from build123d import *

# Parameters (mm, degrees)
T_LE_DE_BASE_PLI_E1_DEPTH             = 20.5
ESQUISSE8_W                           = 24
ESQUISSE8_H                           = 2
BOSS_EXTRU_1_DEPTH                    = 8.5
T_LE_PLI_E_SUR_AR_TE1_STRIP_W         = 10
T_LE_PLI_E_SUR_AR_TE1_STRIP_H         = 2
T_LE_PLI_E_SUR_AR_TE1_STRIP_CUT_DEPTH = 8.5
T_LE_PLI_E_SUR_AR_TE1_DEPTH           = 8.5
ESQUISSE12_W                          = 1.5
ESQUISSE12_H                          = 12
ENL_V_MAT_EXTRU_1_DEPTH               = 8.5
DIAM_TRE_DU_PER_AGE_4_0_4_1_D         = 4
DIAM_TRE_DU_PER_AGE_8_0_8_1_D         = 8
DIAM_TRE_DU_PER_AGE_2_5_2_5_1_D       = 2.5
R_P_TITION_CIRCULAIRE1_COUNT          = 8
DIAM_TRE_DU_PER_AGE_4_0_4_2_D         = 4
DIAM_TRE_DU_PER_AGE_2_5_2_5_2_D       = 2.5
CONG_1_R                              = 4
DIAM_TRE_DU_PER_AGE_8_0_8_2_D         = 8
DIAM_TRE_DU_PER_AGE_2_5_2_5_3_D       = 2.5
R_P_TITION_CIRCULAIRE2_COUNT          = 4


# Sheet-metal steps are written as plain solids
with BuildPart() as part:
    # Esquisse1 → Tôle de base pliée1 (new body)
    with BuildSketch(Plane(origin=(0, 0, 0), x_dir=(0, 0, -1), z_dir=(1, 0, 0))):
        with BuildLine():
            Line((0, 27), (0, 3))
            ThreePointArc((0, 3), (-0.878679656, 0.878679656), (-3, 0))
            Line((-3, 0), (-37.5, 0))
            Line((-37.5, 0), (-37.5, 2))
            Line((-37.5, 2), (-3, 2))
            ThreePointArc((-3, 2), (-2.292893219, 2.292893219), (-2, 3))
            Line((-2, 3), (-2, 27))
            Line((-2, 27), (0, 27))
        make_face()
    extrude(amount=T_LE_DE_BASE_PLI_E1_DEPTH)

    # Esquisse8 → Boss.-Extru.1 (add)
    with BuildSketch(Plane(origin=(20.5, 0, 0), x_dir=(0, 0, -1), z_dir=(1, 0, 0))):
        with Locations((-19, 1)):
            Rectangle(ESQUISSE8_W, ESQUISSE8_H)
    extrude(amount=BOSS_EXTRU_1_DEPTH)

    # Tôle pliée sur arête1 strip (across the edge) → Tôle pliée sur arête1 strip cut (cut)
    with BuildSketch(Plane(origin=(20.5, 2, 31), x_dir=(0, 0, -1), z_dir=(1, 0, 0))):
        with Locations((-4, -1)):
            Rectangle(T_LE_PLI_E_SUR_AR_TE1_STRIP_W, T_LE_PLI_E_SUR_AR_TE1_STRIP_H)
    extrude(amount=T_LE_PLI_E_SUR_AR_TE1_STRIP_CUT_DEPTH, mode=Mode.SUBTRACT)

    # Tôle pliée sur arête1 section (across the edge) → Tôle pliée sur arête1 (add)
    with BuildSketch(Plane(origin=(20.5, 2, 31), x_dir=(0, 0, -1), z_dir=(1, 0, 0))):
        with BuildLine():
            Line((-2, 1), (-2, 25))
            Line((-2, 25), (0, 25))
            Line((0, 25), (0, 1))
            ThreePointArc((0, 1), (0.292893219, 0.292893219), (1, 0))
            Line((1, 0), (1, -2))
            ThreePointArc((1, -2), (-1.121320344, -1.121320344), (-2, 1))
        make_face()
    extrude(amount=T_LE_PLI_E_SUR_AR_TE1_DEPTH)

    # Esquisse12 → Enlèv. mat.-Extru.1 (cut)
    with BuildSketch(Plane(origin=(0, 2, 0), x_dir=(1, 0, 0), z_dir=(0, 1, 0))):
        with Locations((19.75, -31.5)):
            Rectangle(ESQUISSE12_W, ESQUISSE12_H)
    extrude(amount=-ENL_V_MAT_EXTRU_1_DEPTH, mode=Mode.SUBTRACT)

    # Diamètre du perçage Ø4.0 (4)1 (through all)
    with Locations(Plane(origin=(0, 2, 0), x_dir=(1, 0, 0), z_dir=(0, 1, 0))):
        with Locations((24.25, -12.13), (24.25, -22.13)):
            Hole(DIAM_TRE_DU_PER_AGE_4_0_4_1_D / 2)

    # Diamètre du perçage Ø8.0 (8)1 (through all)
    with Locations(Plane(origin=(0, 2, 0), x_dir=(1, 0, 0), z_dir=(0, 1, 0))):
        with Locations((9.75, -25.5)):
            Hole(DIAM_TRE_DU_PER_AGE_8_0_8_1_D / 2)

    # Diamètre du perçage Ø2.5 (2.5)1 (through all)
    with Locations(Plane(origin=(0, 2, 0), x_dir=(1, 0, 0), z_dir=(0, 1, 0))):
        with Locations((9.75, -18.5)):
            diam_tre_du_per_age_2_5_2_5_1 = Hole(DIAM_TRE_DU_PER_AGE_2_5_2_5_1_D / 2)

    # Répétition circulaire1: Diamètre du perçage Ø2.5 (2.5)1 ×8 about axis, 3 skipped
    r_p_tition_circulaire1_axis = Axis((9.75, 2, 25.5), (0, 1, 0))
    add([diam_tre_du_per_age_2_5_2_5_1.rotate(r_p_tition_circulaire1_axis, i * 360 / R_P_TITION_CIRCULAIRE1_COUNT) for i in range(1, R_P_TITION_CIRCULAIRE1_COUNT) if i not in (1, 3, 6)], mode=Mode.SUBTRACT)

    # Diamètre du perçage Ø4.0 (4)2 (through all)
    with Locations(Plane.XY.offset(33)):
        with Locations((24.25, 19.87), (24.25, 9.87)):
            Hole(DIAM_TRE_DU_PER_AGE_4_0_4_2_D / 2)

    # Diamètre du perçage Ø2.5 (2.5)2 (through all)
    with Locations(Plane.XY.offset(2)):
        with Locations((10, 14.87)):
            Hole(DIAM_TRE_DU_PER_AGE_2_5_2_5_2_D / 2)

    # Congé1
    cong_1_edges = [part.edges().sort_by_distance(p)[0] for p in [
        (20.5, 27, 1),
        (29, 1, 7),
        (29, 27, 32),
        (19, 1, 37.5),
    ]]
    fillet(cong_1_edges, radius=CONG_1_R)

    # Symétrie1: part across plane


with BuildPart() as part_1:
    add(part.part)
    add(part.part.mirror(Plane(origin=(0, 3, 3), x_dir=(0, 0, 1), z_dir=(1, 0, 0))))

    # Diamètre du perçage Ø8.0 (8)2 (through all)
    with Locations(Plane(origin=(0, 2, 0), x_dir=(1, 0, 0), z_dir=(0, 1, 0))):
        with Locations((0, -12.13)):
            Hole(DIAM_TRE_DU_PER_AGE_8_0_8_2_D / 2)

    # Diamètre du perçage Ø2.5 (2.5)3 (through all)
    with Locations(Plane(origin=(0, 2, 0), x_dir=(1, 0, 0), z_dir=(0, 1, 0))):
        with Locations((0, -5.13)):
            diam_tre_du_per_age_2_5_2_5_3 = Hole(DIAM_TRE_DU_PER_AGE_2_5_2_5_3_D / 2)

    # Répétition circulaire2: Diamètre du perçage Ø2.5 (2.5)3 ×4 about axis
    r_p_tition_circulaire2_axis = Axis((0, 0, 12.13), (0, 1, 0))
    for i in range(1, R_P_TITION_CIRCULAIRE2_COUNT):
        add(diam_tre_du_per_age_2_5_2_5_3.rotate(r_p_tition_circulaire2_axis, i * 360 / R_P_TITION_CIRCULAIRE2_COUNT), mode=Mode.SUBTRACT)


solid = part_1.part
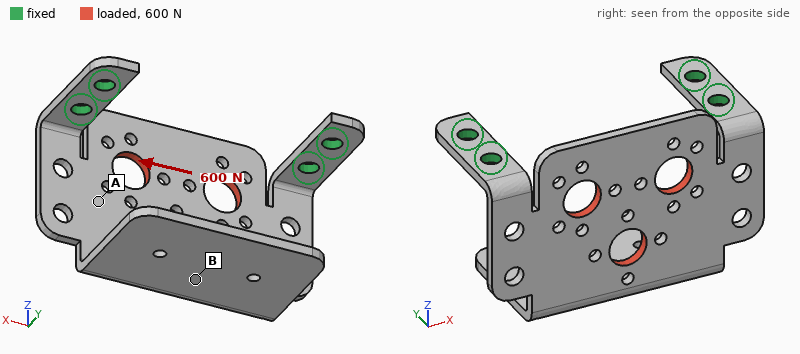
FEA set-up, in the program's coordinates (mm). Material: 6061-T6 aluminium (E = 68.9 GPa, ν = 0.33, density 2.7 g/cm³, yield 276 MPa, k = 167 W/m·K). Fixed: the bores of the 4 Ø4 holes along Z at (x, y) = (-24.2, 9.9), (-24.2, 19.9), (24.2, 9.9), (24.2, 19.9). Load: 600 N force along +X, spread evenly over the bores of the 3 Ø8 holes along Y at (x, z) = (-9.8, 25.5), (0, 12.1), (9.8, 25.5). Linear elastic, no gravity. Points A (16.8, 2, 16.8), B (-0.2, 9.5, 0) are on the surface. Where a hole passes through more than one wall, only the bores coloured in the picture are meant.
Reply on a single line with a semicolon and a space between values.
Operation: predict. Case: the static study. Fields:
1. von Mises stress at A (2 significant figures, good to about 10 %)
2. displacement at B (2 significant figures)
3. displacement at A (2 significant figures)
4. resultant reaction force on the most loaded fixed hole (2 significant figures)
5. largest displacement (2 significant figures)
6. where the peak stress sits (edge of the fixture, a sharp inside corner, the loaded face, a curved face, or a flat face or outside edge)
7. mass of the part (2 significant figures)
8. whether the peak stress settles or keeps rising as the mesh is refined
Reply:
24 MPa; 0.11 mm; 0.079 mm; 380 N; 0.17 mm; edge of the fixture; 16 g; keeps rising
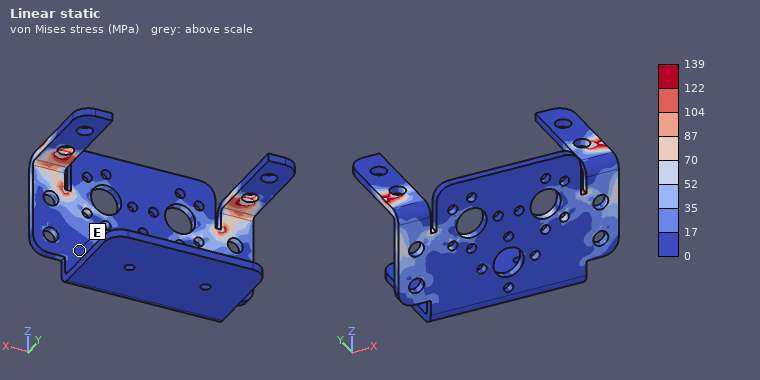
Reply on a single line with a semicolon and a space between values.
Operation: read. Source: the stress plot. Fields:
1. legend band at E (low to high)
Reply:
0 to 17 MPa
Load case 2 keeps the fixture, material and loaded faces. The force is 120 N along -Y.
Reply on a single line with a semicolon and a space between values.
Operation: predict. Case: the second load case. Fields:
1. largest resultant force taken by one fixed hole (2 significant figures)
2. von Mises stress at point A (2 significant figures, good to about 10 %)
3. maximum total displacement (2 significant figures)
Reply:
61 N; 20 MPa; 0.83 mm
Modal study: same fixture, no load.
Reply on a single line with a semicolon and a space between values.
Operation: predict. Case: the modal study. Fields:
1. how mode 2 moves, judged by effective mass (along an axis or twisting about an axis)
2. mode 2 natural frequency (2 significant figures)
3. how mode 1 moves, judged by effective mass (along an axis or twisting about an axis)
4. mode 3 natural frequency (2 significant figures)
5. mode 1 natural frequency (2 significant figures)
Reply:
along X; 1100 Hz; along Y; 1400 Hz; 370 Hz
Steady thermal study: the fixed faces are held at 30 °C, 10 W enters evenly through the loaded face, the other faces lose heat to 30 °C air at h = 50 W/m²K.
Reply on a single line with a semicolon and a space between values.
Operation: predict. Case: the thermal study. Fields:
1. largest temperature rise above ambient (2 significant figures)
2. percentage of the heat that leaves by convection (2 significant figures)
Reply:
25 K; 54 %
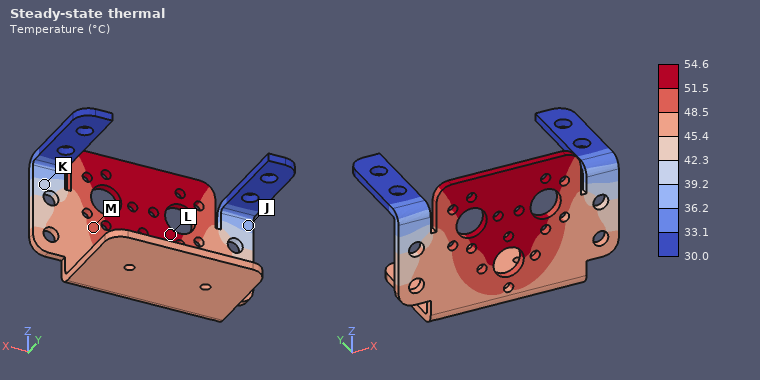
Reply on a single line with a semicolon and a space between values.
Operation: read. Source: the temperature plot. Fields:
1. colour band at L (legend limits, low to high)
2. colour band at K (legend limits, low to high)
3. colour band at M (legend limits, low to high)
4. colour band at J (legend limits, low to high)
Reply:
51.5 to 54.6 °C; 39.2 to 42.3 °C; 48.5 to 51.5 °C; 36.2 to 39.2 °C
